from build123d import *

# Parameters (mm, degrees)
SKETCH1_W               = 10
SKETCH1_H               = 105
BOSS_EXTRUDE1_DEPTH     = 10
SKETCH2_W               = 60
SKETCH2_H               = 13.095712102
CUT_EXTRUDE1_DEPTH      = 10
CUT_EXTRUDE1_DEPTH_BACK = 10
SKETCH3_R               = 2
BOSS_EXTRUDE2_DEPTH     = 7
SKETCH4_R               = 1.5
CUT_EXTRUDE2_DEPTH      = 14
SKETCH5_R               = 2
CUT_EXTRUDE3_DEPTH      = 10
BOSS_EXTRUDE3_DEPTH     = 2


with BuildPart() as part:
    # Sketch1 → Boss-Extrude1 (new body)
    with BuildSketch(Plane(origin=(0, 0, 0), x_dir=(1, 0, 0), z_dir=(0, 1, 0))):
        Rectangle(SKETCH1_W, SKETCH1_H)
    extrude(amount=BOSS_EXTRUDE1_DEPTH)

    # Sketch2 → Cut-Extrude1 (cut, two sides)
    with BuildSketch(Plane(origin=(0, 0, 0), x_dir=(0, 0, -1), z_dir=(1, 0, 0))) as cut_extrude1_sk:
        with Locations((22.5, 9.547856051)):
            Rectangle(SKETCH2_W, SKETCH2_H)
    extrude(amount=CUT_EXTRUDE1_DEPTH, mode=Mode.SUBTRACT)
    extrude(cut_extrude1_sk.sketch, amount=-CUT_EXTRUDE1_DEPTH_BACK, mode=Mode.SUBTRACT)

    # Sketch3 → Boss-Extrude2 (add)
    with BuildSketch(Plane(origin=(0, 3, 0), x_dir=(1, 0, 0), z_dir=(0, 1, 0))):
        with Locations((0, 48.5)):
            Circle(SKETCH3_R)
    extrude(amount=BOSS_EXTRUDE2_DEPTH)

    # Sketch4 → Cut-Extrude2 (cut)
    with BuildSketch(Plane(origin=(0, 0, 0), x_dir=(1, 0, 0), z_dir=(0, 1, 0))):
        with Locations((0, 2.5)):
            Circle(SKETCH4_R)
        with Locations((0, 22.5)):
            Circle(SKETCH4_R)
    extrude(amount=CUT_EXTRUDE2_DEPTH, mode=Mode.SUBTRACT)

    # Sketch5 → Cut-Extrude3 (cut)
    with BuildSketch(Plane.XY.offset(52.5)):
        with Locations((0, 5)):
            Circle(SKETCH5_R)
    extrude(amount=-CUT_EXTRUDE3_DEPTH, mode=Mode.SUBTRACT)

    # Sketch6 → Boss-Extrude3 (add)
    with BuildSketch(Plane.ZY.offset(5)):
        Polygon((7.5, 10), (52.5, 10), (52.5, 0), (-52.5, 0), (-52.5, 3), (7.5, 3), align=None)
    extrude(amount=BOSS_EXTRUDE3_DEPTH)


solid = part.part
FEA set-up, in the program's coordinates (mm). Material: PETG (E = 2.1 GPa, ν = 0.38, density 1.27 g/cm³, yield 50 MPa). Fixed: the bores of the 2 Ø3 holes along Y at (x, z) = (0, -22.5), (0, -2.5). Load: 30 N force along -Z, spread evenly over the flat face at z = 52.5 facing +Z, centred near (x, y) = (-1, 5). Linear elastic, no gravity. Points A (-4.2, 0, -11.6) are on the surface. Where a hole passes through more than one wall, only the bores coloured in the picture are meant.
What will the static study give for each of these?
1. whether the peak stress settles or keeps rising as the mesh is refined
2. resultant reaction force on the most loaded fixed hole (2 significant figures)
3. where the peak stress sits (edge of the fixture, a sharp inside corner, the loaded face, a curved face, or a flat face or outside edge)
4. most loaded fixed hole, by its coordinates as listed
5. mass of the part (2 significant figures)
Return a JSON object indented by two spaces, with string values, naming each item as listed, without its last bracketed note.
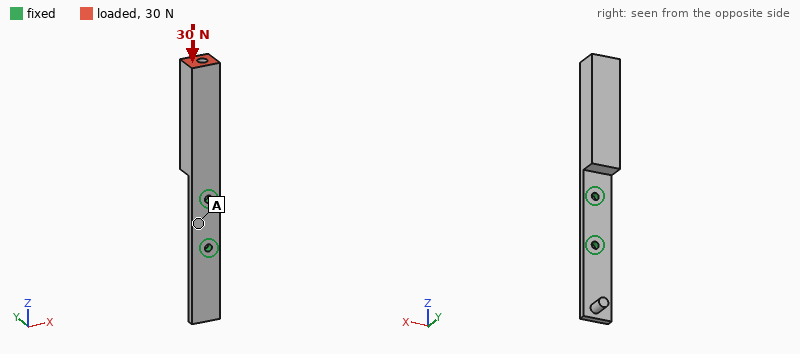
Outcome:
{
  "whether the peak stress settles or keeps rising as the mesh is refined": "keeps rising",
  "resultant reaction force on the most loaded fixed hole": "27 N",
  "where the peak stress sits": "edge of the fixture",
  "most loaded fixed hole, by its coordinates as listed": "(0, -2.5)",
  "mass of the part": "9.5 g"
}
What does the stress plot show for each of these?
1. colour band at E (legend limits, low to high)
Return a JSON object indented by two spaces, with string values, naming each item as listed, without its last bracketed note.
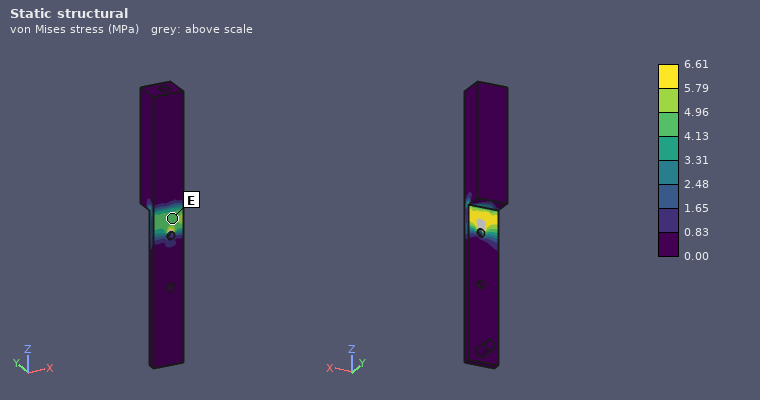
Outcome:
{
  "colour band at E": "4.13 to 4.96 MPa"
}
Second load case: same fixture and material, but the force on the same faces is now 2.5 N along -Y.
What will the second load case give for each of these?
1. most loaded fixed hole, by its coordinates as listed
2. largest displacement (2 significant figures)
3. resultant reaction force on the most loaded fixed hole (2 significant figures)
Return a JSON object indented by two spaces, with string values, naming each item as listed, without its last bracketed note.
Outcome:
{
  "most loaded fixed hole, by its coordinates as listed": "(0, -2.5)",
  "largest displacement": "1.2 mm",
  "resultant reaction force on the most loaded fixed hole": "3.3 N"
}
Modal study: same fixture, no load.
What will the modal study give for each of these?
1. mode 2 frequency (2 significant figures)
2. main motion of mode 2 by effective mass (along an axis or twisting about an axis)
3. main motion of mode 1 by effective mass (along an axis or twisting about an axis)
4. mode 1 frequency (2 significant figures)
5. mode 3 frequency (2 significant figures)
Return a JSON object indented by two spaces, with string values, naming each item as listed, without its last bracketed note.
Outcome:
{
  "mode 2 frequency": "410 Hz",
  "main motion of mode 2 by effective mass": "along X",
  "main motion of mode 1 by effective mass": "along Y",
  "mode 1 frequency": "150 Hz",
  "mode 3 frequency": "640 Hz"
}
